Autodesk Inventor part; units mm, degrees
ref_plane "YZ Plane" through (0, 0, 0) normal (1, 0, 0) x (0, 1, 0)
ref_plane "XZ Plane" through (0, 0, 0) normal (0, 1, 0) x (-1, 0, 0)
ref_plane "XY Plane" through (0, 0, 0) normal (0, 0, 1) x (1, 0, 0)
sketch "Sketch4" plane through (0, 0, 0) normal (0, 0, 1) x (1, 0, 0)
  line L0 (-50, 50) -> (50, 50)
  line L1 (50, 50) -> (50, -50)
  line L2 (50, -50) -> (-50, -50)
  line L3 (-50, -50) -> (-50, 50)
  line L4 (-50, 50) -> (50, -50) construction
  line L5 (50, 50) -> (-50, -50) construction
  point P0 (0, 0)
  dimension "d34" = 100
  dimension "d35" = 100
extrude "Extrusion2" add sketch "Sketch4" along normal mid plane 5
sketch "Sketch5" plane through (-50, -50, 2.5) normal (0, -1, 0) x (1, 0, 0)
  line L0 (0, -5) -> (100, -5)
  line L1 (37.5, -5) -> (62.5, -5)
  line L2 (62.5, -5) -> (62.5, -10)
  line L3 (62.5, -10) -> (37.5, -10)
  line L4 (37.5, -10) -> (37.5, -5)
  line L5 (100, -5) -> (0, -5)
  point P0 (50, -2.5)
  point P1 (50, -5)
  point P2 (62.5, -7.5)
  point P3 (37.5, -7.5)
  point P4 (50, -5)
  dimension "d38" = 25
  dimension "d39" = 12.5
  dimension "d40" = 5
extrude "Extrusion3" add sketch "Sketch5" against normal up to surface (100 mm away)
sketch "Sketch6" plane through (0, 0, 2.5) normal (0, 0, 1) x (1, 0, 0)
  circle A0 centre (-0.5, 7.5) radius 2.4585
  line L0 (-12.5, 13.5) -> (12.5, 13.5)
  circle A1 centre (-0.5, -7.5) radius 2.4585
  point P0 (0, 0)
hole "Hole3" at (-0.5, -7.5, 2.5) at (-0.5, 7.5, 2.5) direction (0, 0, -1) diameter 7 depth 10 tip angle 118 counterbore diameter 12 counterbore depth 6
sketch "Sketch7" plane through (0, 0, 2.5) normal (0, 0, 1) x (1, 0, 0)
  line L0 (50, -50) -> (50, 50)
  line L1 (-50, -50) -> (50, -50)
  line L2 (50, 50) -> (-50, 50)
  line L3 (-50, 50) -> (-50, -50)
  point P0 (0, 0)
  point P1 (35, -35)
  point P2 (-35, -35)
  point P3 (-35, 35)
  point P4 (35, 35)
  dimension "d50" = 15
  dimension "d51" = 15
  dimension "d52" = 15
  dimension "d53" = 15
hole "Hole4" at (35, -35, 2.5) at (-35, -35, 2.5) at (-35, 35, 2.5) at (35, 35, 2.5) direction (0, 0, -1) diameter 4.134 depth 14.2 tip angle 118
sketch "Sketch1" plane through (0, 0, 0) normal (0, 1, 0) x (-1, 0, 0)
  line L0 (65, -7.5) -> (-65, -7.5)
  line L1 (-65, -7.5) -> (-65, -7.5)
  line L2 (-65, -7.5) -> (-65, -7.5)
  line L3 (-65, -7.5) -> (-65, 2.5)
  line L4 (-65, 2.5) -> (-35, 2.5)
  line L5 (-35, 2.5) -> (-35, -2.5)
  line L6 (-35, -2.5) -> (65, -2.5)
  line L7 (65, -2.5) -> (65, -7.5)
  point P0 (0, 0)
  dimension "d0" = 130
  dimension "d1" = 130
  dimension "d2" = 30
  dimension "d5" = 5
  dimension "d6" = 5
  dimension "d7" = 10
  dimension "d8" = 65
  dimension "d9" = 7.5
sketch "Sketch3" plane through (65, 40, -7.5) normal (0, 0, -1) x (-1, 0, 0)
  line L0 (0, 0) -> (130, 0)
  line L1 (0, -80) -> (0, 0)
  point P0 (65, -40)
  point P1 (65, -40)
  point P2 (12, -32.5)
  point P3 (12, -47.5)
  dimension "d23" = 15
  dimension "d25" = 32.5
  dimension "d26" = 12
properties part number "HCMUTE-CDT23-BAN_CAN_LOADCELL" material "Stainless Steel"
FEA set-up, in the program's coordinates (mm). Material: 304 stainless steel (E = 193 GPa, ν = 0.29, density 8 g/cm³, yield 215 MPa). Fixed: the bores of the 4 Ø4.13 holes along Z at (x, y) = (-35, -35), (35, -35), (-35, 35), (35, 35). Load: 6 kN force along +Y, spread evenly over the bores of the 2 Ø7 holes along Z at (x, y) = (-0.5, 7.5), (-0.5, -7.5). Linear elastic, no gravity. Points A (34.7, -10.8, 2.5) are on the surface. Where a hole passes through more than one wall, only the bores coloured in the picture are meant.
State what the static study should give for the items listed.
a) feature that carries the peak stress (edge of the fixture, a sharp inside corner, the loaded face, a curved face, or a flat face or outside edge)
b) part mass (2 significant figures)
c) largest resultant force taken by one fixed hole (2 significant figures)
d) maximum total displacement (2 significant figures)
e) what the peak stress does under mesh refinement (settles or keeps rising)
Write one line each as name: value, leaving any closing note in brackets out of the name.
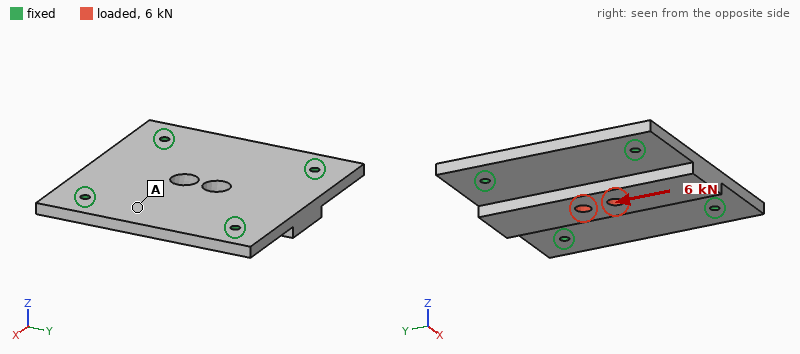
feature that carries the peak stress: edge of the fixture
part mass: 480 g
largest resultant force taken by one fixed hole: 1.6 kN
maximum total displacement: 9.7 µm
what the peak stress does under mesh refinement: keeps rising
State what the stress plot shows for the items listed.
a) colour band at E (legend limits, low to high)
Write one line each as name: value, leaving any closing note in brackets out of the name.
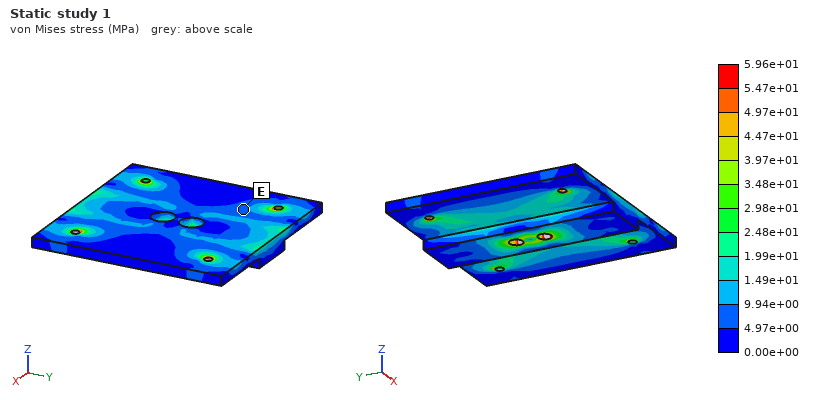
colour band at E: 4.97e+00 to 9.94e+00 MPa
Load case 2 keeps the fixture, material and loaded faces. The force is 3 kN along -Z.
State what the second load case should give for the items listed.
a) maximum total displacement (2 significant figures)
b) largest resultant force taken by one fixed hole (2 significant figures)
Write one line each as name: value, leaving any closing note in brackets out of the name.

maximum total displacement: 43 µm
largest resultant force taken by one fixed hole: 1.0 kN
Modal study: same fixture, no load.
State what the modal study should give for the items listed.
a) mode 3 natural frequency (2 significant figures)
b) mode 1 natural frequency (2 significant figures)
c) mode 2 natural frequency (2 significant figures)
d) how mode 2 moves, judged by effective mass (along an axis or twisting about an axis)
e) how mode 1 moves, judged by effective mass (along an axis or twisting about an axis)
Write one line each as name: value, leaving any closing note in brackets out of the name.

mode 3 natural frequency: 5200 Hz
mode 1 natural frequency: 3600 Hz
mode 2 natural frequency: 4700 Hz
how mode 2 moves, judged by effective mass: twisting about X
how mode 1 moves, judged by effective mass: along Z
